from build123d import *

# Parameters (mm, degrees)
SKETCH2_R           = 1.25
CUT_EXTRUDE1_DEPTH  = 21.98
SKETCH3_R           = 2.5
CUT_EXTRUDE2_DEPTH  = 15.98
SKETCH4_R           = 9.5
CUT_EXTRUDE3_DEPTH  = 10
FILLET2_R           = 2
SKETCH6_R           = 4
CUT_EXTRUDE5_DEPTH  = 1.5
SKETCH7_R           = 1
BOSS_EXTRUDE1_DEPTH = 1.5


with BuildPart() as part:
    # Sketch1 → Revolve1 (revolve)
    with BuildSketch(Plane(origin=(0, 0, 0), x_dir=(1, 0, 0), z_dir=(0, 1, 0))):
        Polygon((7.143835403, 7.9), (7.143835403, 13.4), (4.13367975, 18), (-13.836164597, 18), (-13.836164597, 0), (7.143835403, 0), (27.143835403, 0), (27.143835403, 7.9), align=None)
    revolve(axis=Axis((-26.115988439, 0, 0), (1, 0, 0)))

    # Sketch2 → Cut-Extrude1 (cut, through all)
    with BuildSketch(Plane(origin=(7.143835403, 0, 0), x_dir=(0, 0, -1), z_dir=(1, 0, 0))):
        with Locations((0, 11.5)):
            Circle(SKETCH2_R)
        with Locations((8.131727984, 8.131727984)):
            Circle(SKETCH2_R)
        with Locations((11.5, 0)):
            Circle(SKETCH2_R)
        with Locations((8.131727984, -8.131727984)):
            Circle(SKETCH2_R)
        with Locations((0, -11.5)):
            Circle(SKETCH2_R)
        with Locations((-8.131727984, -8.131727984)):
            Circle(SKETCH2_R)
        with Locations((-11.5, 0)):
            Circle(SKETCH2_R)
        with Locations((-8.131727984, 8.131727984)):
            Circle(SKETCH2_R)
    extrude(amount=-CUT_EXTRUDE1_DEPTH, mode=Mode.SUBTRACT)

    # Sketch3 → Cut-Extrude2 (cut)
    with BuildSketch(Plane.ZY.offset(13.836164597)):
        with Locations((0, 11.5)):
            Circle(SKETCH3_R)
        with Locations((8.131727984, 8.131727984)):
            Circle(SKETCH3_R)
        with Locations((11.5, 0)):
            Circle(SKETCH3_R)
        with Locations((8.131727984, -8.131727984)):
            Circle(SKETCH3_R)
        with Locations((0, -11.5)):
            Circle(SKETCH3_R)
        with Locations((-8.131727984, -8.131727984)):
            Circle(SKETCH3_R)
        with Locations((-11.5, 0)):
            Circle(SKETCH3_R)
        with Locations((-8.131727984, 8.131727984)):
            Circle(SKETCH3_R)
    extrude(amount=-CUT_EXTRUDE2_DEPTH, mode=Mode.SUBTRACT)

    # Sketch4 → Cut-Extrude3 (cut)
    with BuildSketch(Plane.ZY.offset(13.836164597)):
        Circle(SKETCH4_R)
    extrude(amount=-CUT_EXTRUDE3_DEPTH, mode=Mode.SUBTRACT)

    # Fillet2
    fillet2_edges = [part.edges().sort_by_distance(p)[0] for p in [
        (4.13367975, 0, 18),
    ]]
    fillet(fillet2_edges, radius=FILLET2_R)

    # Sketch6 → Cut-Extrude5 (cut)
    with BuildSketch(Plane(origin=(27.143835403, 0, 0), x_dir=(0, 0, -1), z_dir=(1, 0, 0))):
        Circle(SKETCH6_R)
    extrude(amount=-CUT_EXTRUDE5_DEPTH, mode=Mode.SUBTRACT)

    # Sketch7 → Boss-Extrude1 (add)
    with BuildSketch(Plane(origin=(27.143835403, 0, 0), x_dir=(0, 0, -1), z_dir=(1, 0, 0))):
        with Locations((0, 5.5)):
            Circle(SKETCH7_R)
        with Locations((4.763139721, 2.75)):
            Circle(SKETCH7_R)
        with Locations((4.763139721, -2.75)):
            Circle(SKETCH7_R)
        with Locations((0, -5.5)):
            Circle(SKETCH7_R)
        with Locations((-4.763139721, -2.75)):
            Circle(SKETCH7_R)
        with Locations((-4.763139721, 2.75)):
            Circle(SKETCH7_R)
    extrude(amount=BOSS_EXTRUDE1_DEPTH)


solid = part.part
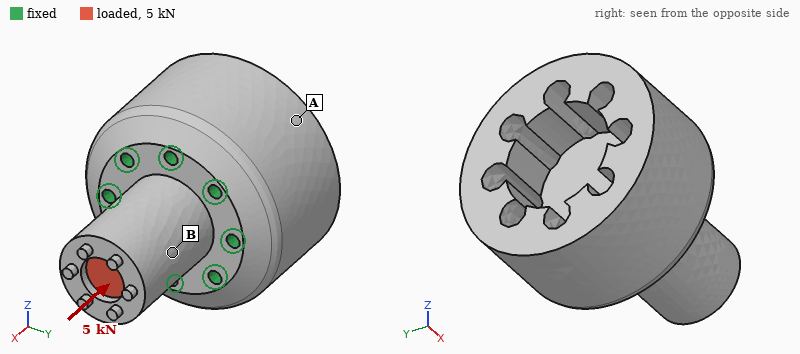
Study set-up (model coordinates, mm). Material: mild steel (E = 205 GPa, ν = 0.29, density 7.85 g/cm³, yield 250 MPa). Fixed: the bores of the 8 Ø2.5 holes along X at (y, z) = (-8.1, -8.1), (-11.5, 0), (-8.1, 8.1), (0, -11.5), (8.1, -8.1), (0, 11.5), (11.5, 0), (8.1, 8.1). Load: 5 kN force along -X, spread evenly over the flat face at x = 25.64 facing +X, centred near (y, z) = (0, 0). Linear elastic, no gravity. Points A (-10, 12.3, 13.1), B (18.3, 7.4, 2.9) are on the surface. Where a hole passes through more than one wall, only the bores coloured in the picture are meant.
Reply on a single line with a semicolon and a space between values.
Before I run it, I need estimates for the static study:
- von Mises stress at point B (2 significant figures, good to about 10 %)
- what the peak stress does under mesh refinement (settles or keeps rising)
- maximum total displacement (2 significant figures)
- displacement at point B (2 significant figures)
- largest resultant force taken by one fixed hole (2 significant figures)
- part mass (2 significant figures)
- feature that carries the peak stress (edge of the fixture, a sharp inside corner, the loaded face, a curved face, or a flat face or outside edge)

20 MPa; keeps rising; 5.0 µm; 2.4 µm; 630 N; 150 g; edge of the fixture
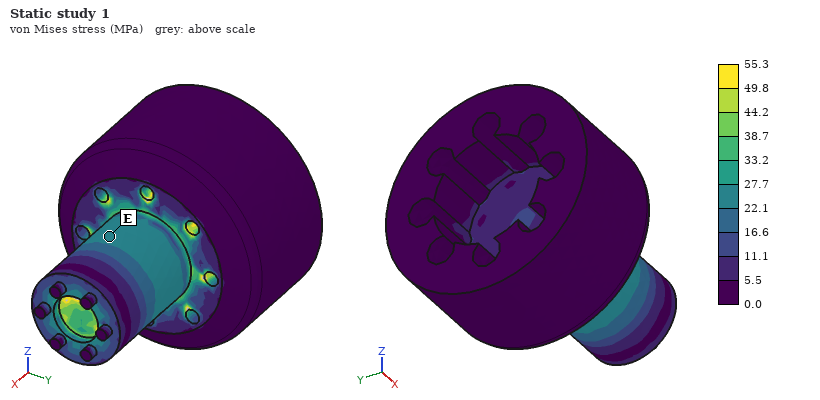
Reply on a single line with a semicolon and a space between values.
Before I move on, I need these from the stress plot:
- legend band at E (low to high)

22.1 to 27.7 MPa
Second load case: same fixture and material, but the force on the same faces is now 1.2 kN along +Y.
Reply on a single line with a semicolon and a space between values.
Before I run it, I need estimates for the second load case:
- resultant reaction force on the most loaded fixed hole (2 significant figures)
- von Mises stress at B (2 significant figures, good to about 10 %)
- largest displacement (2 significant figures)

620 N; 22 MPa; 10 µm
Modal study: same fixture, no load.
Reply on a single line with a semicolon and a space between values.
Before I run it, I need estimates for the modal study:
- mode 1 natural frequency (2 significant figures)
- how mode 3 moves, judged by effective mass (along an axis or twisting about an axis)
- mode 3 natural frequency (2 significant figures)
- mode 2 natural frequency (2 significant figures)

17 kHz; along Z; 23 kHz; 17 kHz
